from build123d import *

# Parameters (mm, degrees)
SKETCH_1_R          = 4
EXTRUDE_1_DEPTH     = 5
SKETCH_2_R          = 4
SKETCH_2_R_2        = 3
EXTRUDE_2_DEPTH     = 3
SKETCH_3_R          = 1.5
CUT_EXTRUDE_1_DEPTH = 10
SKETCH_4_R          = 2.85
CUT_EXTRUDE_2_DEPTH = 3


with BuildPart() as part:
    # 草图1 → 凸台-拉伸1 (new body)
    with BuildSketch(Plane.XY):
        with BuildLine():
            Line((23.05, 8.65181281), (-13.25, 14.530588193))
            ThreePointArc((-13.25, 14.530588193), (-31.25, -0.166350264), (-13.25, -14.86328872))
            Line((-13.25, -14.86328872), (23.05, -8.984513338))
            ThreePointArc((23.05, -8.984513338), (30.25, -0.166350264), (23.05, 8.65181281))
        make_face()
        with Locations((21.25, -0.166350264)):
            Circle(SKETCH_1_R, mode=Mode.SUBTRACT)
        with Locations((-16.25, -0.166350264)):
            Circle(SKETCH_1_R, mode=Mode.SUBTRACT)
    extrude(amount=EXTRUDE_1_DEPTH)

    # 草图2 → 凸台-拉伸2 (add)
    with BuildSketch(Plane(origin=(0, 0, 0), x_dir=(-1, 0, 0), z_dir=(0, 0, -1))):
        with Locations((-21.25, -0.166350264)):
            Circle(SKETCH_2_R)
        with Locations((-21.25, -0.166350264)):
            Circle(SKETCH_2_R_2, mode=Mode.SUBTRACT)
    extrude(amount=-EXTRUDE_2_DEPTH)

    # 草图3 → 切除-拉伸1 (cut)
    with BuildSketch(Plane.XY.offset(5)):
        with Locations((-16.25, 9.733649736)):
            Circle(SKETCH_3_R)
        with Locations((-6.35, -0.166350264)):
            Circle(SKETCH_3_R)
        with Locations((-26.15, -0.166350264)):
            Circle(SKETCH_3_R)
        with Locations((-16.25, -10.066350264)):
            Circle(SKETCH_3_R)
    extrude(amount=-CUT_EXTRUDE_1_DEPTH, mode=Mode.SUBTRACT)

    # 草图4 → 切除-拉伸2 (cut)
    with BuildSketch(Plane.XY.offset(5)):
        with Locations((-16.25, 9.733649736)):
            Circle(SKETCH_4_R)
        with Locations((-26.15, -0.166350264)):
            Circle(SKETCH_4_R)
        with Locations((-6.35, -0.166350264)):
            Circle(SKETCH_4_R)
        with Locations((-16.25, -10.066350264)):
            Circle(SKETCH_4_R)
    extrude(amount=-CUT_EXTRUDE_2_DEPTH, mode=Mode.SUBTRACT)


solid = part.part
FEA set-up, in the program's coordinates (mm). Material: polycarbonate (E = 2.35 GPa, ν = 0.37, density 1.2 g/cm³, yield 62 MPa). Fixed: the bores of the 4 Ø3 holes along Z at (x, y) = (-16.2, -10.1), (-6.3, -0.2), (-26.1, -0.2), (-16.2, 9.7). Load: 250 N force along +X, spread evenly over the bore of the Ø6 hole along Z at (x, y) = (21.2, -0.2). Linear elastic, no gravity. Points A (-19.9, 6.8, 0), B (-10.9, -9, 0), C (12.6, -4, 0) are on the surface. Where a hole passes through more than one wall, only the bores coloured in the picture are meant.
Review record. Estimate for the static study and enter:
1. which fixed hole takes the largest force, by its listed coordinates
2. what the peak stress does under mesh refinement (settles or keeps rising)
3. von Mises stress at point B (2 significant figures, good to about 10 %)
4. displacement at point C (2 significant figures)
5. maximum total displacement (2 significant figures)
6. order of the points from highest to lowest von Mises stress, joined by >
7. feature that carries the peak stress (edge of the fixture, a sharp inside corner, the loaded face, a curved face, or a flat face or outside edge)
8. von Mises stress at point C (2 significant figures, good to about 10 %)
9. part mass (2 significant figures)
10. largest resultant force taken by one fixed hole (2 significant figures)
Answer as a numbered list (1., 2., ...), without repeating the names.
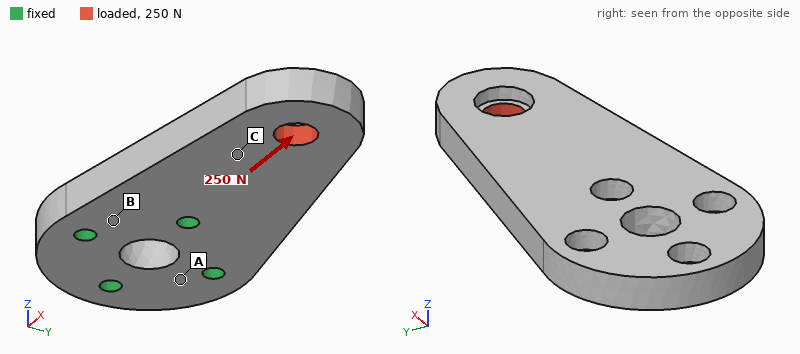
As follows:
1. (-6.3, -0.2)
2. keeps rising
3. 2.7 MPa
4. 0.076 mm
5. 0.27 mm
6. C > B > A
7. edge of the fixture
8. 5.5 MPa
9. 7.4 g
10. 130 N
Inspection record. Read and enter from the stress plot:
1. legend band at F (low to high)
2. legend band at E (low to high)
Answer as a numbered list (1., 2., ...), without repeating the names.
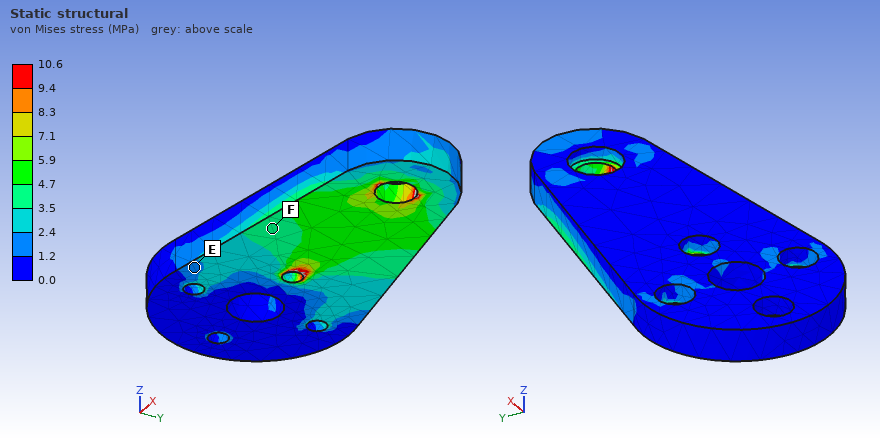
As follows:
1. 3.5 to 4.7 MPa
2. 1.2 to 2.4 MPa
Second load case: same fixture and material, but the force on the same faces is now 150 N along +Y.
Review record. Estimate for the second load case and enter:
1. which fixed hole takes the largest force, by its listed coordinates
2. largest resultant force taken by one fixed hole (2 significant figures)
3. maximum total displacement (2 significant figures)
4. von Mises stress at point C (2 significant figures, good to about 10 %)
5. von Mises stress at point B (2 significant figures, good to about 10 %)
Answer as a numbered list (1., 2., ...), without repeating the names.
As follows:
1. (-6.3, -0.2)
2. 180 N
3. 0.30 mm
4. 4.4 MPa
5. 6.7 MPa
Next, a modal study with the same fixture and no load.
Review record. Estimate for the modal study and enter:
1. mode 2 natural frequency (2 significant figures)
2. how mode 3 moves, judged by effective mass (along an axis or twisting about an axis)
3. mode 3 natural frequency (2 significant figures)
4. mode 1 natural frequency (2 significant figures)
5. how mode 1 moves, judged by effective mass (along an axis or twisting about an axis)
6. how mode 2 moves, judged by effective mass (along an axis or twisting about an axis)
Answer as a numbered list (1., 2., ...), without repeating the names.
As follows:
1. 2700 Hz
2. along Y
3. 3100 Hz
4. 910 Hz
5. along Z
6. twisting about X
